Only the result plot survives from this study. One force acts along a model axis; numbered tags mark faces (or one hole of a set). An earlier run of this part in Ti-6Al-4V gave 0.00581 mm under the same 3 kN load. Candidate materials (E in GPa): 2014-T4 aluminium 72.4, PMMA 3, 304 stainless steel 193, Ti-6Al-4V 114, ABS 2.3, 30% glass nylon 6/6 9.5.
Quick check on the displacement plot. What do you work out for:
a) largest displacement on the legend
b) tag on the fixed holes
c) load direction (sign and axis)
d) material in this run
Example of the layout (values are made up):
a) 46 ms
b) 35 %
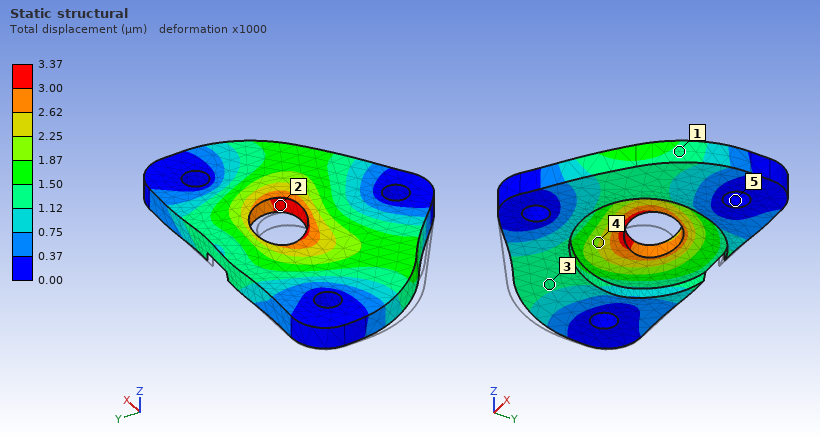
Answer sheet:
a) 3.37 µm
b) 5
c) +X
d) 304 stainless steel
